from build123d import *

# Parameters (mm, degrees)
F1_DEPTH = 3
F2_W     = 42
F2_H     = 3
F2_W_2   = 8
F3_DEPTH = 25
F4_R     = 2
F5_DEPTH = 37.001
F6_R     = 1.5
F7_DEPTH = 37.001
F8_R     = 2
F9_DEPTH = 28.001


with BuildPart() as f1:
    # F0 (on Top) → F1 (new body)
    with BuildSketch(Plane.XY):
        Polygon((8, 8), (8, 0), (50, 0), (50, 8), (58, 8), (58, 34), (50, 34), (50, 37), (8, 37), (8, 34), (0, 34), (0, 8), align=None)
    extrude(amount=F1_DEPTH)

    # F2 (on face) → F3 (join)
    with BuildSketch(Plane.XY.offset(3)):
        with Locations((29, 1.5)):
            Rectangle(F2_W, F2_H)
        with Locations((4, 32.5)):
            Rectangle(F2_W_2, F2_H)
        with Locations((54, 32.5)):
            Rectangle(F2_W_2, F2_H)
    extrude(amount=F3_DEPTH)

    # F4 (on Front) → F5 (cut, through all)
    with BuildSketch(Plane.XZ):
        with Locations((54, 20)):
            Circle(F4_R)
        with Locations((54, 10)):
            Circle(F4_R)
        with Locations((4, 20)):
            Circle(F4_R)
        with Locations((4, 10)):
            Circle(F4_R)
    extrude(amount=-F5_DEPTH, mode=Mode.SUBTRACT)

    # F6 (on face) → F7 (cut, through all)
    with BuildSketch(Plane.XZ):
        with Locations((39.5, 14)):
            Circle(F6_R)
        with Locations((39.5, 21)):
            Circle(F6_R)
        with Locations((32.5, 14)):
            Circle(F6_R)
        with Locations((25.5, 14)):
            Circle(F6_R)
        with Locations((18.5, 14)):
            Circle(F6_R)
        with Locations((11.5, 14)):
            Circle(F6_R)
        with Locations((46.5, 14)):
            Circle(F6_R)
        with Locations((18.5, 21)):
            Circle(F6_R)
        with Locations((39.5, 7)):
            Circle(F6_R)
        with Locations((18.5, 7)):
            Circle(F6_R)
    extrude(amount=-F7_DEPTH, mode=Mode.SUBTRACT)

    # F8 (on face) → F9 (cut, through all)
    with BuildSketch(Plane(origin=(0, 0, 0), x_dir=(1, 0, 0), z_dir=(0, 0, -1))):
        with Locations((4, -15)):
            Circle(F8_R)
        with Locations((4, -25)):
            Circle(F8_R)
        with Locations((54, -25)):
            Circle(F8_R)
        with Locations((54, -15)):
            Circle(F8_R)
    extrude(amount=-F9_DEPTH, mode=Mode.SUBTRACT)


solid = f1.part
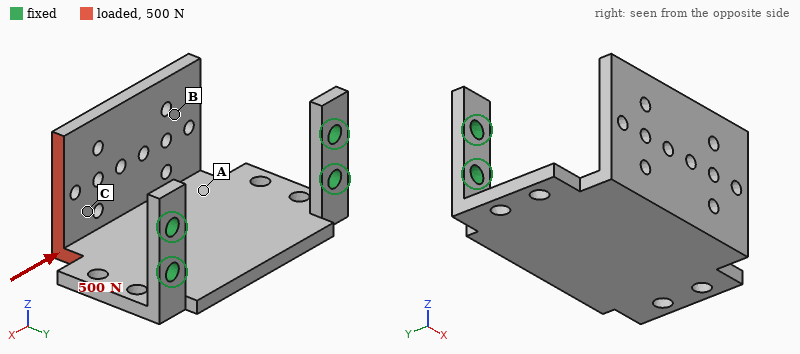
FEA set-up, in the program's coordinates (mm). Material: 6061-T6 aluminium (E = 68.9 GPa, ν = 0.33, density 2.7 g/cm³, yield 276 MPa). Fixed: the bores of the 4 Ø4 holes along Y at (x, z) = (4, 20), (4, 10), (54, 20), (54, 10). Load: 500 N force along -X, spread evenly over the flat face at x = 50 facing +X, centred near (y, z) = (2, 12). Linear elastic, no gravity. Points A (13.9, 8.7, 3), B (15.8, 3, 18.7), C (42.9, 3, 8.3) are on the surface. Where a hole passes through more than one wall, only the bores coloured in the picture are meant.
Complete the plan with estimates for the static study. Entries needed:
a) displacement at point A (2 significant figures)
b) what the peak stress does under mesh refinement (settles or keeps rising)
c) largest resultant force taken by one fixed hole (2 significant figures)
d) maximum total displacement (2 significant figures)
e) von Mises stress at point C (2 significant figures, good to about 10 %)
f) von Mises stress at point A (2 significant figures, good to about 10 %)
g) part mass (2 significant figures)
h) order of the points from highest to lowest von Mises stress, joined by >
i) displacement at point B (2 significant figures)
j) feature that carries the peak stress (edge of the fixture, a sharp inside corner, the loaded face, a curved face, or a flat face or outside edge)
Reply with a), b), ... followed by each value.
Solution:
a) 0.14 mm
b) keeps rising
c) 420 N
d) 0.42 mm
e) 34 MPa
f) 63 MPa
g) 26 g
h) A > C > B
i) 0.28 mm
j) edge of the fixture
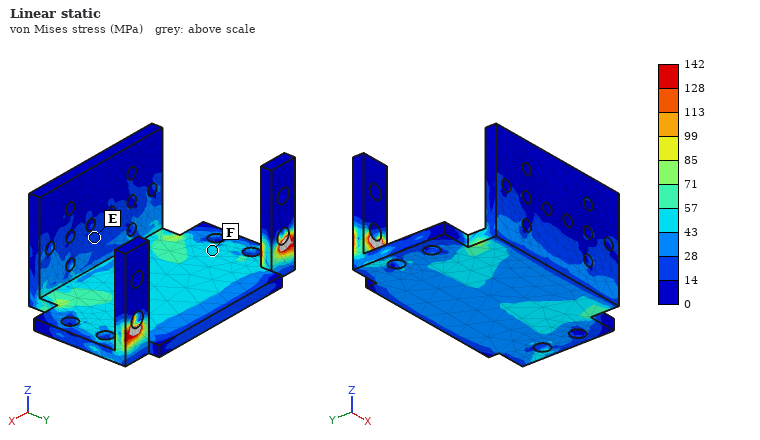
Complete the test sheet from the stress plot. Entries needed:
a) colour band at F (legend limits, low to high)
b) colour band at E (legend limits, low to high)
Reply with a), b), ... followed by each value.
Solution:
a) 43 to 57 MPa
b) 14 to 28 MPa
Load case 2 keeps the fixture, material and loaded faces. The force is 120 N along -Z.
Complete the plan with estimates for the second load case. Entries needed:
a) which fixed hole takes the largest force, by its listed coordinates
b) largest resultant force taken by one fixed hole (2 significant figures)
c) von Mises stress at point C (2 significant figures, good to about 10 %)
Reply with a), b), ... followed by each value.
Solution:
a) (54, 10)
b) 110 N
c) 16 MPa
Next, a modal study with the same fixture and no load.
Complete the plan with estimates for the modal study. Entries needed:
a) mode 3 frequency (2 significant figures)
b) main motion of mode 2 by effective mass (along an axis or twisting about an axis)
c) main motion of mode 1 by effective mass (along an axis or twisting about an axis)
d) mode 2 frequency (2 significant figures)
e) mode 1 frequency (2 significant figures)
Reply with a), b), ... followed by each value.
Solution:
a) 2300 Hz
b) along X
c) along Z
d) 1700 Hz
e) 620 Hz
